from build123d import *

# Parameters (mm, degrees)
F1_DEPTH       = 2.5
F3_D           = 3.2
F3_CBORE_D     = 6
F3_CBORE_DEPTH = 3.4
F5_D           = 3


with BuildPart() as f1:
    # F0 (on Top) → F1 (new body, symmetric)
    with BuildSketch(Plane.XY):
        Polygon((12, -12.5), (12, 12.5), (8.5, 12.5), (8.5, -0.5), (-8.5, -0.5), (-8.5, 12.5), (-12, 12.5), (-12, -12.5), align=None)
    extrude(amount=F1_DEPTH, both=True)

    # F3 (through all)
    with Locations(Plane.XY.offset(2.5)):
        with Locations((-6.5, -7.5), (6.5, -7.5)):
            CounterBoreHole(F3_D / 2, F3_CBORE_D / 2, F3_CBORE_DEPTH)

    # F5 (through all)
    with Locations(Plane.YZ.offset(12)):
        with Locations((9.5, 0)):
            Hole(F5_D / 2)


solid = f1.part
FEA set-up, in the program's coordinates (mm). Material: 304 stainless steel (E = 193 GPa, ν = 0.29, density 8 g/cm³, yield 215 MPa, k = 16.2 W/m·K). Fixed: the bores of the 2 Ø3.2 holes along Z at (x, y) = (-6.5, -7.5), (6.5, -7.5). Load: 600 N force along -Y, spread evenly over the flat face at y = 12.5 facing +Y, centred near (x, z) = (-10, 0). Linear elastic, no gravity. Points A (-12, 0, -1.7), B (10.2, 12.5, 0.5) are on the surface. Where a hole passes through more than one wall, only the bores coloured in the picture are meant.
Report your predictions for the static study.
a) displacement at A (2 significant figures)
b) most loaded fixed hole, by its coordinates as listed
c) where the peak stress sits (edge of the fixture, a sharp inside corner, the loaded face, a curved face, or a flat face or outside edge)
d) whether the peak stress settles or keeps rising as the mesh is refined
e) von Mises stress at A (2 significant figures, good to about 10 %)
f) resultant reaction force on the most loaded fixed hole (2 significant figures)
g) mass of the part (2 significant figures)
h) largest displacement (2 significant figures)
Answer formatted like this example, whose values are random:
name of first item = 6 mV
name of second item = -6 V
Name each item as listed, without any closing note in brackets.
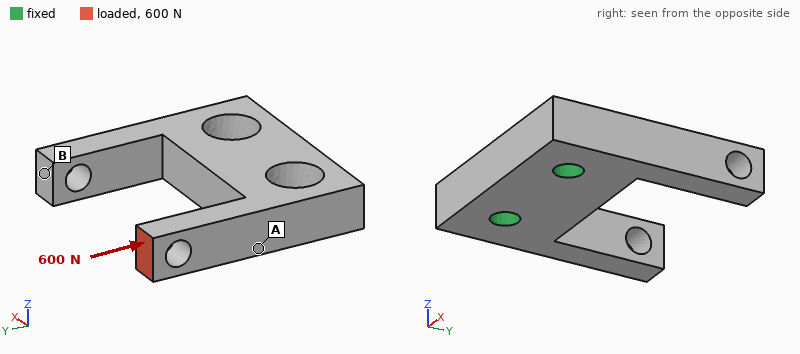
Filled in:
displacement at A = 6.1 µm
most loaded fixed hole, by its coordinates as listed = (-6.5, -7.5)
where the peak stress sits = edge of the fixture
whether the peak stress settles or keeps rising as the mesh is refined = keeps rising
von Mises stress at A = 37 MPa
resultant reaction force on the most loaded fixed hole = 700 N
mass of the part = 13 g
largest displacement = 17 µm
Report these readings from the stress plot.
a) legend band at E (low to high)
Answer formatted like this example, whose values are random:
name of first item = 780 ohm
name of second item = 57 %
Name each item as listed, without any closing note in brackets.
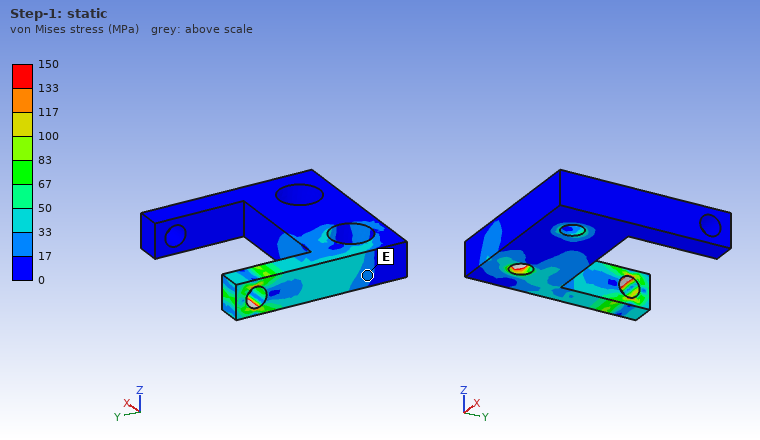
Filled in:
legend band at E = 17 to 33 MPa
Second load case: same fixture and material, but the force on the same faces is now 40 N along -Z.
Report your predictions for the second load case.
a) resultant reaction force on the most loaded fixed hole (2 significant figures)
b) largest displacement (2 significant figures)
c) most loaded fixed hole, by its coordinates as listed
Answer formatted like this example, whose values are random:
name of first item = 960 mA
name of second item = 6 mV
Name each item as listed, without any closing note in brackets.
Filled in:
resultant reaction force on the most loaded fixed hole = 53 N
largest displacement = 19 µm
most loaded fixed hole, by its coordinates as listed = (-6.5, -7.5)
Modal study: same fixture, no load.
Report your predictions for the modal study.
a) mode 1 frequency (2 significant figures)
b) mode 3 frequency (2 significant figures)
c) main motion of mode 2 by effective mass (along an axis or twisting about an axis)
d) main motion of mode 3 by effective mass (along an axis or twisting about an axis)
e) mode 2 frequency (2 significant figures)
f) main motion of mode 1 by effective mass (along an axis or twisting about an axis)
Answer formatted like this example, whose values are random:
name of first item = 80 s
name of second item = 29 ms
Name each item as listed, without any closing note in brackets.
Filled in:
mode 1 frequency = 8200 Hz
mode 3 frequency = 12 kHz
main motion of mode 2 by effective mass = twisting about Y
main motion of mode 3 by effective mass = along X
mode 2 frequency = 10 kHz
main motion of mode 1 by effective mass = along Z
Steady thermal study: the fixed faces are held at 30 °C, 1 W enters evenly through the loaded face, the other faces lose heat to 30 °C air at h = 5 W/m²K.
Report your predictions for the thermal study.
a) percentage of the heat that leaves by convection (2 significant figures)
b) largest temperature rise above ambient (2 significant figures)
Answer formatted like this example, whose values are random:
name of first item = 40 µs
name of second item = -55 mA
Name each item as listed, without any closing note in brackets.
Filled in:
percentage of the heat that leaves by convection = 6.8 %
largest temperature rise above ambient = 76 K
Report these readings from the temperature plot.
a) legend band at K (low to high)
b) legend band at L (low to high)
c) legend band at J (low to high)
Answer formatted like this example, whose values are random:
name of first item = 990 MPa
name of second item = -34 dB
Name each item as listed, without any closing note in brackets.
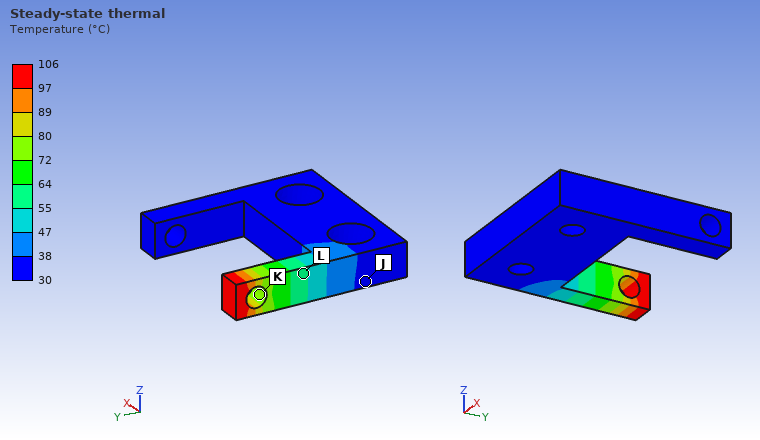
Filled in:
legend band at K = 72 to 80 °C
legend band at L = 55 to 64 °C
legend band at J = 30 to 38 °C
